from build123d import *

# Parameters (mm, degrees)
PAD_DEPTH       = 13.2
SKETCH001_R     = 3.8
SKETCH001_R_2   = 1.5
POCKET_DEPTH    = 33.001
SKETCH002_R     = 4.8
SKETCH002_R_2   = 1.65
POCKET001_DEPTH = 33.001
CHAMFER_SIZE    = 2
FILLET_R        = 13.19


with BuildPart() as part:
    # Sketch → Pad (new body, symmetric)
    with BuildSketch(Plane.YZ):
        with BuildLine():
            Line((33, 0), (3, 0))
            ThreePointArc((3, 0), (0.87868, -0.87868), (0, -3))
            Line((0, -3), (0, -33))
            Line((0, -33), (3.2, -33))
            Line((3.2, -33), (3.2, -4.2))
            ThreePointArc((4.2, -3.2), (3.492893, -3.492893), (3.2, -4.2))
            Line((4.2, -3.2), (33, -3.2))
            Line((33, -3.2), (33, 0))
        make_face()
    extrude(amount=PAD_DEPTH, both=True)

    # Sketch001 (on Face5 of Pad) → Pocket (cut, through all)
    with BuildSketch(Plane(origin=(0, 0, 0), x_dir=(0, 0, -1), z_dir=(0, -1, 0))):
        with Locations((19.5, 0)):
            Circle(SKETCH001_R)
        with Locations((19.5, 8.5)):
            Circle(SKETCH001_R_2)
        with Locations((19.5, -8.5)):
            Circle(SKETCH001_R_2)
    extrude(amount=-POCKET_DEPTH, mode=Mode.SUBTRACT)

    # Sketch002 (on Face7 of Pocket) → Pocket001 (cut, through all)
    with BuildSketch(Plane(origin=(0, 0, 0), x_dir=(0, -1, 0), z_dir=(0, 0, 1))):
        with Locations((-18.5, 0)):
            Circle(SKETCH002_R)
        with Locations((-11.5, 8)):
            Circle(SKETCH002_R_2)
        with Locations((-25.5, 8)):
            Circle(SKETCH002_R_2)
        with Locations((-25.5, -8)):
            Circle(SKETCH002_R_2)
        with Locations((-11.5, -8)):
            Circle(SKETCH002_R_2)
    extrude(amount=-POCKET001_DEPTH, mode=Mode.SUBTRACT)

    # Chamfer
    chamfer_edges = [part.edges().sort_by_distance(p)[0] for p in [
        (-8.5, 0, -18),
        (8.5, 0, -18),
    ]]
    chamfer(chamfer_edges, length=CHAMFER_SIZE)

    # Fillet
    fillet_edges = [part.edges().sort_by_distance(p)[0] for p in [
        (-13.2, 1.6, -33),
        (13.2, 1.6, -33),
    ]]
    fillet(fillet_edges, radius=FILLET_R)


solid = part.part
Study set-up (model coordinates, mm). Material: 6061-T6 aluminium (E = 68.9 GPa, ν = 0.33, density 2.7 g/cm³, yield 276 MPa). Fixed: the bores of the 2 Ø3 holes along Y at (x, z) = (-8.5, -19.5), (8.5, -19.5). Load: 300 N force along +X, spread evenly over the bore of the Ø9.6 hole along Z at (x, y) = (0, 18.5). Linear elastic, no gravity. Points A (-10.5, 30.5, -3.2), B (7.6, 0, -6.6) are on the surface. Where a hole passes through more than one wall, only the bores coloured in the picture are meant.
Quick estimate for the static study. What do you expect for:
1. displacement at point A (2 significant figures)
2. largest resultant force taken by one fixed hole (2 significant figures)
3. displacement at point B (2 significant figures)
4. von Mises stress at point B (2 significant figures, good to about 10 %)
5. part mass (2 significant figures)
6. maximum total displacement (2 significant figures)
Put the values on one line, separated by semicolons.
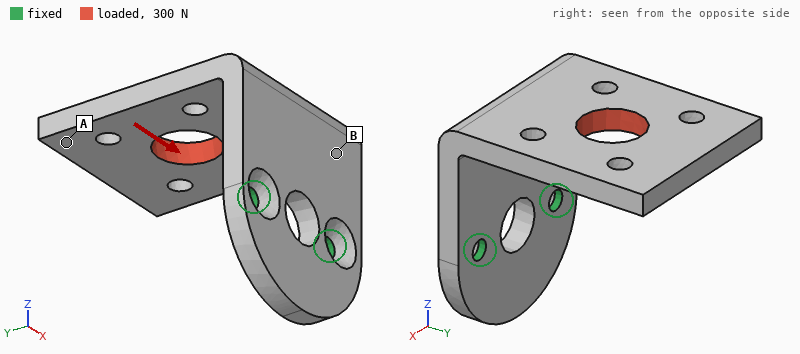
0.28 mm; 400 N; 0.050 mm; 65 MPa; 12 g; 0.31 mm
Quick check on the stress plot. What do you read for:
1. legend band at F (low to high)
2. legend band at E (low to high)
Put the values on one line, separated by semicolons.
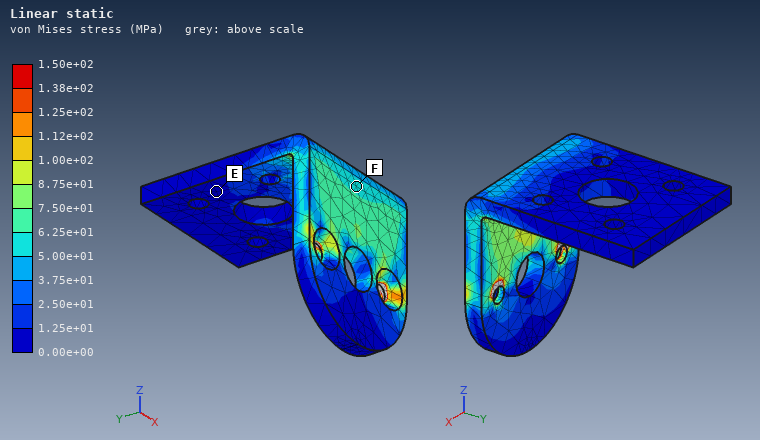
5.00e+01 to 6.25e+01 MPa; 0.00e+00 to 1.25e+01 MPa
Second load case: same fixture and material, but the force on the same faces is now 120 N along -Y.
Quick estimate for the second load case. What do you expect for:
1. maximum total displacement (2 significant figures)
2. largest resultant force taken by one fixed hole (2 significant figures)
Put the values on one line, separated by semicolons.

0.24 mm; 64 N
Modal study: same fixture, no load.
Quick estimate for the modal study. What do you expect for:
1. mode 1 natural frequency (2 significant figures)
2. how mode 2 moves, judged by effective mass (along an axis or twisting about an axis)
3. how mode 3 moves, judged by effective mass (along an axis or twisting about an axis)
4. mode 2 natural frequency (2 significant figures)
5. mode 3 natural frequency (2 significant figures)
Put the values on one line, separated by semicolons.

1200 Hz; along X; along Y; 2400 Hz; 3600 Hz
